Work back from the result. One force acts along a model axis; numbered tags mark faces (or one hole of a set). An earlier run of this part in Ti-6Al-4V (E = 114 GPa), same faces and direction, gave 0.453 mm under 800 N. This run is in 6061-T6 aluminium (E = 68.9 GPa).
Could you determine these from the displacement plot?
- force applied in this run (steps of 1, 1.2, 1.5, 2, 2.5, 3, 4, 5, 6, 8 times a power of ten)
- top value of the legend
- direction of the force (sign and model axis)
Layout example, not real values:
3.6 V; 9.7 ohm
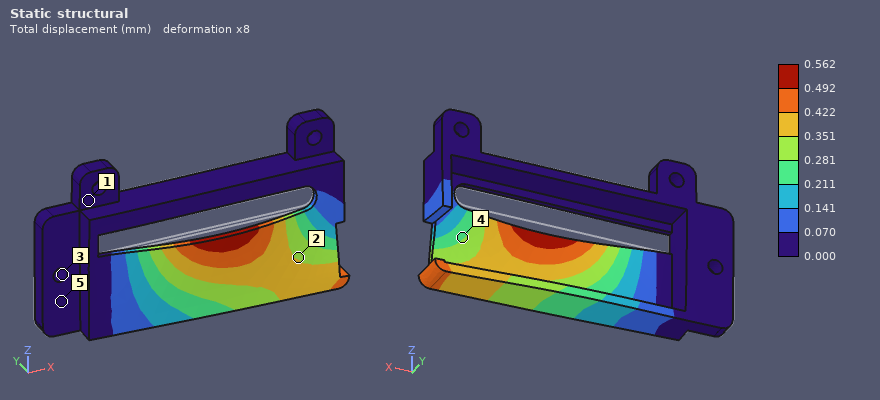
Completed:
600 N; 0.562 mm; -Y
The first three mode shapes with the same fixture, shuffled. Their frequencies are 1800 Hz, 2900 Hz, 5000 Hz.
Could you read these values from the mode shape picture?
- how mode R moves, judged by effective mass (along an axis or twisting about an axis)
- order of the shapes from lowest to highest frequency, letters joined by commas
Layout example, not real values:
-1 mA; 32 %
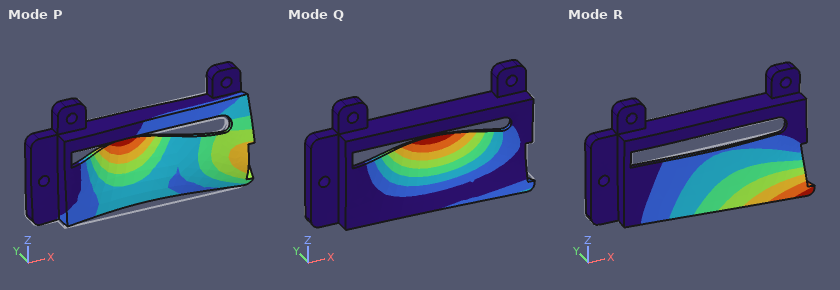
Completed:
along Y; R, Q, P
